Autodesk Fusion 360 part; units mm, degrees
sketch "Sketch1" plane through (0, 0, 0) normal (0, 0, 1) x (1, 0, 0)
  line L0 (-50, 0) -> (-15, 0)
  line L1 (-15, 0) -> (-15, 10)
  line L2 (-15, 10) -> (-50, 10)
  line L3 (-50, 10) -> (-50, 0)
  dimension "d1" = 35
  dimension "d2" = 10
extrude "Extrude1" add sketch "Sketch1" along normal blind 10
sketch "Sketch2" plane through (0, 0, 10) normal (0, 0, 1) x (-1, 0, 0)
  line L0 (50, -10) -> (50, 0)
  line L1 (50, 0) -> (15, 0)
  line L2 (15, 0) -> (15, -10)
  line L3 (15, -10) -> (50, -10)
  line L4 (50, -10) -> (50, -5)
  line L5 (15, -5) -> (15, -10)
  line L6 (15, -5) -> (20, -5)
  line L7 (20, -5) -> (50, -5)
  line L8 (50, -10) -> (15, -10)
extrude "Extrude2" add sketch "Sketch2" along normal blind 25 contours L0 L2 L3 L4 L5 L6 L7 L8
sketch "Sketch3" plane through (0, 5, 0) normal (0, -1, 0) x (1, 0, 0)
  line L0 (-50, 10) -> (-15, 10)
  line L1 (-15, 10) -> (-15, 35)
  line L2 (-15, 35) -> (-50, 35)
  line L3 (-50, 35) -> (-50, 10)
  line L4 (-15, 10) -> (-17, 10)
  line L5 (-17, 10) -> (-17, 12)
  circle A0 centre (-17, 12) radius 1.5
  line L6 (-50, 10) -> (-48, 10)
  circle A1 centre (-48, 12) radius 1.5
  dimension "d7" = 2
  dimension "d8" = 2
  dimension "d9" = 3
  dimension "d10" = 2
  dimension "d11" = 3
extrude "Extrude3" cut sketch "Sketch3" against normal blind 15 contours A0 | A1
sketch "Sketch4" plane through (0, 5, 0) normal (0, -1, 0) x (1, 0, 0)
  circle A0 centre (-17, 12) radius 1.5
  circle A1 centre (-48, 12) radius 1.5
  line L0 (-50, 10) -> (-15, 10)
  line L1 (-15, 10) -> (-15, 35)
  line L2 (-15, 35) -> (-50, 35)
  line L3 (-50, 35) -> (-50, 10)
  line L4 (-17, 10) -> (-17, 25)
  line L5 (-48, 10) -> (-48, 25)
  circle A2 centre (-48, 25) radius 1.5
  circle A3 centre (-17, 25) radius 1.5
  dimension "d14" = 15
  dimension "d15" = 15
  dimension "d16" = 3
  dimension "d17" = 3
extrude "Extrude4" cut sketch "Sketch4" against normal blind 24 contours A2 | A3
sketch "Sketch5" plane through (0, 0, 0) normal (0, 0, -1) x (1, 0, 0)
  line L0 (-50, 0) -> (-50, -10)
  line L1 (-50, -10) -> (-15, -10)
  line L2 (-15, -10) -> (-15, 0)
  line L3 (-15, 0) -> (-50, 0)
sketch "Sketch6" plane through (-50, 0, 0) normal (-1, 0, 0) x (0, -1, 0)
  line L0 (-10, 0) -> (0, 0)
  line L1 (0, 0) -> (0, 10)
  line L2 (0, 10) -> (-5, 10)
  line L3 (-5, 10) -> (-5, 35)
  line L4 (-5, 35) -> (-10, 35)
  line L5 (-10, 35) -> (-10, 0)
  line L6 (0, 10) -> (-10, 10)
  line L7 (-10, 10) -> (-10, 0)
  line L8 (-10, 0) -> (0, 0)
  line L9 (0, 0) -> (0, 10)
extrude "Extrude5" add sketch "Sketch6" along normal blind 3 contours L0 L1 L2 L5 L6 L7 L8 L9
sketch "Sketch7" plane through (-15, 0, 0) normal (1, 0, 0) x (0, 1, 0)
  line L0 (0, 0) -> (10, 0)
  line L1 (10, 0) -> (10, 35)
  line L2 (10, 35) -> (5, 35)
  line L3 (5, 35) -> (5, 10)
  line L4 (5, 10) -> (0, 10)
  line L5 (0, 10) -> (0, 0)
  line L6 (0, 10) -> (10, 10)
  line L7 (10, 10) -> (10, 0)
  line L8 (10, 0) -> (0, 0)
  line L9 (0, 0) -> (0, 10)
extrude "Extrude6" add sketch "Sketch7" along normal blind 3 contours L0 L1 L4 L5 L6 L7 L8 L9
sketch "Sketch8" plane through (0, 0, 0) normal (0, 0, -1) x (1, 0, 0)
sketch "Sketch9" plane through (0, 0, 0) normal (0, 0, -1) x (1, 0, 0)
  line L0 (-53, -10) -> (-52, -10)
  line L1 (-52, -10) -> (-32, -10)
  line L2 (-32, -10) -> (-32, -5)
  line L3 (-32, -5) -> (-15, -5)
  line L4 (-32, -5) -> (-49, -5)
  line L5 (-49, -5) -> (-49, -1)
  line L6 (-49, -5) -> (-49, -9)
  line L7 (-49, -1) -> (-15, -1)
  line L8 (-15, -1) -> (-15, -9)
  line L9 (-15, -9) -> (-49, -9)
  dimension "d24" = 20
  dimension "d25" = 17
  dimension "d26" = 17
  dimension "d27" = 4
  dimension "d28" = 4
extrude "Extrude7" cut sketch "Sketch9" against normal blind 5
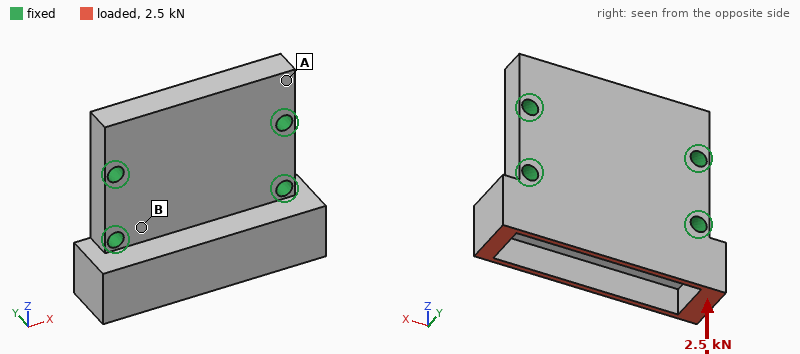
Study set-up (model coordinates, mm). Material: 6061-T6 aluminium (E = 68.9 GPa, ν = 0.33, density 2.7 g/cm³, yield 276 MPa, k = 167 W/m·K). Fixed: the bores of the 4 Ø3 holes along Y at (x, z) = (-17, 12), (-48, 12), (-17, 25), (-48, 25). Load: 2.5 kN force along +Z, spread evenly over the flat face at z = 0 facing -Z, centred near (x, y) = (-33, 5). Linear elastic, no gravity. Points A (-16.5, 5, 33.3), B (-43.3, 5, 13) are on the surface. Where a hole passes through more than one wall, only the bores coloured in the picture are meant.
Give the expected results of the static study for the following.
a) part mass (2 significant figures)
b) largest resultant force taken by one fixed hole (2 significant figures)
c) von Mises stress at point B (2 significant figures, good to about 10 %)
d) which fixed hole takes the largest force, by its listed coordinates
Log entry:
19 g
1.2 kN
23 MPa
(-48, 12)
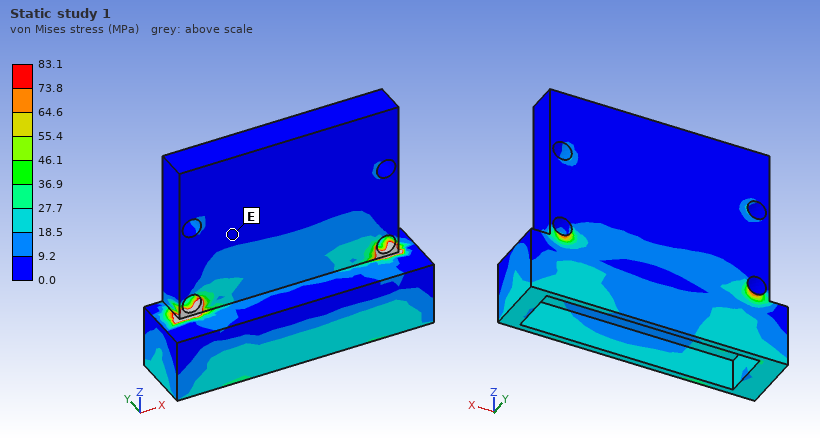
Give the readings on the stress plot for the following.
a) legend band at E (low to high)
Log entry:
0.0 to 9.2 MPa
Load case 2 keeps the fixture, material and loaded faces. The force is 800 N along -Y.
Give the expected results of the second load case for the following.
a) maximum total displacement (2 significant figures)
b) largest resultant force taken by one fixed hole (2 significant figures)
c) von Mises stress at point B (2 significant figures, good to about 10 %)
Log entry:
72 µm
530 N
27 MPa
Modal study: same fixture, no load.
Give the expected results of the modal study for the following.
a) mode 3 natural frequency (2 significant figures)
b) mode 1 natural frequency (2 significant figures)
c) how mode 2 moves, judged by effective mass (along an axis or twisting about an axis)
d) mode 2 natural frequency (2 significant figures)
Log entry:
22 kHz
17 kHz
along Y
20 kHz
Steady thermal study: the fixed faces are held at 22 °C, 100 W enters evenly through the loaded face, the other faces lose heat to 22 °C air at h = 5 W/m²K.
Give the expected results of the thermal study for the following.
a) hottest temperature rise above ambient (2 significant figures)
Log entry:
57 K
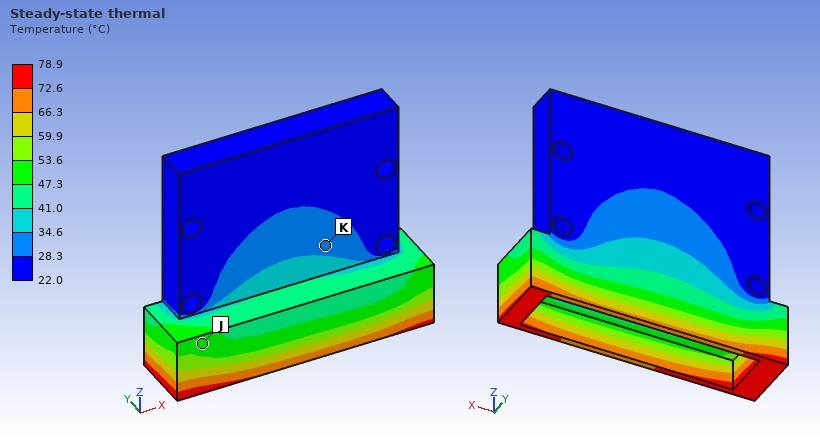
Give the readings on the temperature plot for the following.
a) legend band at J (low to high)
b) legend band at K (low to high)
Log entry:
47.3 to 53.6 °C
28.3 to 34.6 °C
